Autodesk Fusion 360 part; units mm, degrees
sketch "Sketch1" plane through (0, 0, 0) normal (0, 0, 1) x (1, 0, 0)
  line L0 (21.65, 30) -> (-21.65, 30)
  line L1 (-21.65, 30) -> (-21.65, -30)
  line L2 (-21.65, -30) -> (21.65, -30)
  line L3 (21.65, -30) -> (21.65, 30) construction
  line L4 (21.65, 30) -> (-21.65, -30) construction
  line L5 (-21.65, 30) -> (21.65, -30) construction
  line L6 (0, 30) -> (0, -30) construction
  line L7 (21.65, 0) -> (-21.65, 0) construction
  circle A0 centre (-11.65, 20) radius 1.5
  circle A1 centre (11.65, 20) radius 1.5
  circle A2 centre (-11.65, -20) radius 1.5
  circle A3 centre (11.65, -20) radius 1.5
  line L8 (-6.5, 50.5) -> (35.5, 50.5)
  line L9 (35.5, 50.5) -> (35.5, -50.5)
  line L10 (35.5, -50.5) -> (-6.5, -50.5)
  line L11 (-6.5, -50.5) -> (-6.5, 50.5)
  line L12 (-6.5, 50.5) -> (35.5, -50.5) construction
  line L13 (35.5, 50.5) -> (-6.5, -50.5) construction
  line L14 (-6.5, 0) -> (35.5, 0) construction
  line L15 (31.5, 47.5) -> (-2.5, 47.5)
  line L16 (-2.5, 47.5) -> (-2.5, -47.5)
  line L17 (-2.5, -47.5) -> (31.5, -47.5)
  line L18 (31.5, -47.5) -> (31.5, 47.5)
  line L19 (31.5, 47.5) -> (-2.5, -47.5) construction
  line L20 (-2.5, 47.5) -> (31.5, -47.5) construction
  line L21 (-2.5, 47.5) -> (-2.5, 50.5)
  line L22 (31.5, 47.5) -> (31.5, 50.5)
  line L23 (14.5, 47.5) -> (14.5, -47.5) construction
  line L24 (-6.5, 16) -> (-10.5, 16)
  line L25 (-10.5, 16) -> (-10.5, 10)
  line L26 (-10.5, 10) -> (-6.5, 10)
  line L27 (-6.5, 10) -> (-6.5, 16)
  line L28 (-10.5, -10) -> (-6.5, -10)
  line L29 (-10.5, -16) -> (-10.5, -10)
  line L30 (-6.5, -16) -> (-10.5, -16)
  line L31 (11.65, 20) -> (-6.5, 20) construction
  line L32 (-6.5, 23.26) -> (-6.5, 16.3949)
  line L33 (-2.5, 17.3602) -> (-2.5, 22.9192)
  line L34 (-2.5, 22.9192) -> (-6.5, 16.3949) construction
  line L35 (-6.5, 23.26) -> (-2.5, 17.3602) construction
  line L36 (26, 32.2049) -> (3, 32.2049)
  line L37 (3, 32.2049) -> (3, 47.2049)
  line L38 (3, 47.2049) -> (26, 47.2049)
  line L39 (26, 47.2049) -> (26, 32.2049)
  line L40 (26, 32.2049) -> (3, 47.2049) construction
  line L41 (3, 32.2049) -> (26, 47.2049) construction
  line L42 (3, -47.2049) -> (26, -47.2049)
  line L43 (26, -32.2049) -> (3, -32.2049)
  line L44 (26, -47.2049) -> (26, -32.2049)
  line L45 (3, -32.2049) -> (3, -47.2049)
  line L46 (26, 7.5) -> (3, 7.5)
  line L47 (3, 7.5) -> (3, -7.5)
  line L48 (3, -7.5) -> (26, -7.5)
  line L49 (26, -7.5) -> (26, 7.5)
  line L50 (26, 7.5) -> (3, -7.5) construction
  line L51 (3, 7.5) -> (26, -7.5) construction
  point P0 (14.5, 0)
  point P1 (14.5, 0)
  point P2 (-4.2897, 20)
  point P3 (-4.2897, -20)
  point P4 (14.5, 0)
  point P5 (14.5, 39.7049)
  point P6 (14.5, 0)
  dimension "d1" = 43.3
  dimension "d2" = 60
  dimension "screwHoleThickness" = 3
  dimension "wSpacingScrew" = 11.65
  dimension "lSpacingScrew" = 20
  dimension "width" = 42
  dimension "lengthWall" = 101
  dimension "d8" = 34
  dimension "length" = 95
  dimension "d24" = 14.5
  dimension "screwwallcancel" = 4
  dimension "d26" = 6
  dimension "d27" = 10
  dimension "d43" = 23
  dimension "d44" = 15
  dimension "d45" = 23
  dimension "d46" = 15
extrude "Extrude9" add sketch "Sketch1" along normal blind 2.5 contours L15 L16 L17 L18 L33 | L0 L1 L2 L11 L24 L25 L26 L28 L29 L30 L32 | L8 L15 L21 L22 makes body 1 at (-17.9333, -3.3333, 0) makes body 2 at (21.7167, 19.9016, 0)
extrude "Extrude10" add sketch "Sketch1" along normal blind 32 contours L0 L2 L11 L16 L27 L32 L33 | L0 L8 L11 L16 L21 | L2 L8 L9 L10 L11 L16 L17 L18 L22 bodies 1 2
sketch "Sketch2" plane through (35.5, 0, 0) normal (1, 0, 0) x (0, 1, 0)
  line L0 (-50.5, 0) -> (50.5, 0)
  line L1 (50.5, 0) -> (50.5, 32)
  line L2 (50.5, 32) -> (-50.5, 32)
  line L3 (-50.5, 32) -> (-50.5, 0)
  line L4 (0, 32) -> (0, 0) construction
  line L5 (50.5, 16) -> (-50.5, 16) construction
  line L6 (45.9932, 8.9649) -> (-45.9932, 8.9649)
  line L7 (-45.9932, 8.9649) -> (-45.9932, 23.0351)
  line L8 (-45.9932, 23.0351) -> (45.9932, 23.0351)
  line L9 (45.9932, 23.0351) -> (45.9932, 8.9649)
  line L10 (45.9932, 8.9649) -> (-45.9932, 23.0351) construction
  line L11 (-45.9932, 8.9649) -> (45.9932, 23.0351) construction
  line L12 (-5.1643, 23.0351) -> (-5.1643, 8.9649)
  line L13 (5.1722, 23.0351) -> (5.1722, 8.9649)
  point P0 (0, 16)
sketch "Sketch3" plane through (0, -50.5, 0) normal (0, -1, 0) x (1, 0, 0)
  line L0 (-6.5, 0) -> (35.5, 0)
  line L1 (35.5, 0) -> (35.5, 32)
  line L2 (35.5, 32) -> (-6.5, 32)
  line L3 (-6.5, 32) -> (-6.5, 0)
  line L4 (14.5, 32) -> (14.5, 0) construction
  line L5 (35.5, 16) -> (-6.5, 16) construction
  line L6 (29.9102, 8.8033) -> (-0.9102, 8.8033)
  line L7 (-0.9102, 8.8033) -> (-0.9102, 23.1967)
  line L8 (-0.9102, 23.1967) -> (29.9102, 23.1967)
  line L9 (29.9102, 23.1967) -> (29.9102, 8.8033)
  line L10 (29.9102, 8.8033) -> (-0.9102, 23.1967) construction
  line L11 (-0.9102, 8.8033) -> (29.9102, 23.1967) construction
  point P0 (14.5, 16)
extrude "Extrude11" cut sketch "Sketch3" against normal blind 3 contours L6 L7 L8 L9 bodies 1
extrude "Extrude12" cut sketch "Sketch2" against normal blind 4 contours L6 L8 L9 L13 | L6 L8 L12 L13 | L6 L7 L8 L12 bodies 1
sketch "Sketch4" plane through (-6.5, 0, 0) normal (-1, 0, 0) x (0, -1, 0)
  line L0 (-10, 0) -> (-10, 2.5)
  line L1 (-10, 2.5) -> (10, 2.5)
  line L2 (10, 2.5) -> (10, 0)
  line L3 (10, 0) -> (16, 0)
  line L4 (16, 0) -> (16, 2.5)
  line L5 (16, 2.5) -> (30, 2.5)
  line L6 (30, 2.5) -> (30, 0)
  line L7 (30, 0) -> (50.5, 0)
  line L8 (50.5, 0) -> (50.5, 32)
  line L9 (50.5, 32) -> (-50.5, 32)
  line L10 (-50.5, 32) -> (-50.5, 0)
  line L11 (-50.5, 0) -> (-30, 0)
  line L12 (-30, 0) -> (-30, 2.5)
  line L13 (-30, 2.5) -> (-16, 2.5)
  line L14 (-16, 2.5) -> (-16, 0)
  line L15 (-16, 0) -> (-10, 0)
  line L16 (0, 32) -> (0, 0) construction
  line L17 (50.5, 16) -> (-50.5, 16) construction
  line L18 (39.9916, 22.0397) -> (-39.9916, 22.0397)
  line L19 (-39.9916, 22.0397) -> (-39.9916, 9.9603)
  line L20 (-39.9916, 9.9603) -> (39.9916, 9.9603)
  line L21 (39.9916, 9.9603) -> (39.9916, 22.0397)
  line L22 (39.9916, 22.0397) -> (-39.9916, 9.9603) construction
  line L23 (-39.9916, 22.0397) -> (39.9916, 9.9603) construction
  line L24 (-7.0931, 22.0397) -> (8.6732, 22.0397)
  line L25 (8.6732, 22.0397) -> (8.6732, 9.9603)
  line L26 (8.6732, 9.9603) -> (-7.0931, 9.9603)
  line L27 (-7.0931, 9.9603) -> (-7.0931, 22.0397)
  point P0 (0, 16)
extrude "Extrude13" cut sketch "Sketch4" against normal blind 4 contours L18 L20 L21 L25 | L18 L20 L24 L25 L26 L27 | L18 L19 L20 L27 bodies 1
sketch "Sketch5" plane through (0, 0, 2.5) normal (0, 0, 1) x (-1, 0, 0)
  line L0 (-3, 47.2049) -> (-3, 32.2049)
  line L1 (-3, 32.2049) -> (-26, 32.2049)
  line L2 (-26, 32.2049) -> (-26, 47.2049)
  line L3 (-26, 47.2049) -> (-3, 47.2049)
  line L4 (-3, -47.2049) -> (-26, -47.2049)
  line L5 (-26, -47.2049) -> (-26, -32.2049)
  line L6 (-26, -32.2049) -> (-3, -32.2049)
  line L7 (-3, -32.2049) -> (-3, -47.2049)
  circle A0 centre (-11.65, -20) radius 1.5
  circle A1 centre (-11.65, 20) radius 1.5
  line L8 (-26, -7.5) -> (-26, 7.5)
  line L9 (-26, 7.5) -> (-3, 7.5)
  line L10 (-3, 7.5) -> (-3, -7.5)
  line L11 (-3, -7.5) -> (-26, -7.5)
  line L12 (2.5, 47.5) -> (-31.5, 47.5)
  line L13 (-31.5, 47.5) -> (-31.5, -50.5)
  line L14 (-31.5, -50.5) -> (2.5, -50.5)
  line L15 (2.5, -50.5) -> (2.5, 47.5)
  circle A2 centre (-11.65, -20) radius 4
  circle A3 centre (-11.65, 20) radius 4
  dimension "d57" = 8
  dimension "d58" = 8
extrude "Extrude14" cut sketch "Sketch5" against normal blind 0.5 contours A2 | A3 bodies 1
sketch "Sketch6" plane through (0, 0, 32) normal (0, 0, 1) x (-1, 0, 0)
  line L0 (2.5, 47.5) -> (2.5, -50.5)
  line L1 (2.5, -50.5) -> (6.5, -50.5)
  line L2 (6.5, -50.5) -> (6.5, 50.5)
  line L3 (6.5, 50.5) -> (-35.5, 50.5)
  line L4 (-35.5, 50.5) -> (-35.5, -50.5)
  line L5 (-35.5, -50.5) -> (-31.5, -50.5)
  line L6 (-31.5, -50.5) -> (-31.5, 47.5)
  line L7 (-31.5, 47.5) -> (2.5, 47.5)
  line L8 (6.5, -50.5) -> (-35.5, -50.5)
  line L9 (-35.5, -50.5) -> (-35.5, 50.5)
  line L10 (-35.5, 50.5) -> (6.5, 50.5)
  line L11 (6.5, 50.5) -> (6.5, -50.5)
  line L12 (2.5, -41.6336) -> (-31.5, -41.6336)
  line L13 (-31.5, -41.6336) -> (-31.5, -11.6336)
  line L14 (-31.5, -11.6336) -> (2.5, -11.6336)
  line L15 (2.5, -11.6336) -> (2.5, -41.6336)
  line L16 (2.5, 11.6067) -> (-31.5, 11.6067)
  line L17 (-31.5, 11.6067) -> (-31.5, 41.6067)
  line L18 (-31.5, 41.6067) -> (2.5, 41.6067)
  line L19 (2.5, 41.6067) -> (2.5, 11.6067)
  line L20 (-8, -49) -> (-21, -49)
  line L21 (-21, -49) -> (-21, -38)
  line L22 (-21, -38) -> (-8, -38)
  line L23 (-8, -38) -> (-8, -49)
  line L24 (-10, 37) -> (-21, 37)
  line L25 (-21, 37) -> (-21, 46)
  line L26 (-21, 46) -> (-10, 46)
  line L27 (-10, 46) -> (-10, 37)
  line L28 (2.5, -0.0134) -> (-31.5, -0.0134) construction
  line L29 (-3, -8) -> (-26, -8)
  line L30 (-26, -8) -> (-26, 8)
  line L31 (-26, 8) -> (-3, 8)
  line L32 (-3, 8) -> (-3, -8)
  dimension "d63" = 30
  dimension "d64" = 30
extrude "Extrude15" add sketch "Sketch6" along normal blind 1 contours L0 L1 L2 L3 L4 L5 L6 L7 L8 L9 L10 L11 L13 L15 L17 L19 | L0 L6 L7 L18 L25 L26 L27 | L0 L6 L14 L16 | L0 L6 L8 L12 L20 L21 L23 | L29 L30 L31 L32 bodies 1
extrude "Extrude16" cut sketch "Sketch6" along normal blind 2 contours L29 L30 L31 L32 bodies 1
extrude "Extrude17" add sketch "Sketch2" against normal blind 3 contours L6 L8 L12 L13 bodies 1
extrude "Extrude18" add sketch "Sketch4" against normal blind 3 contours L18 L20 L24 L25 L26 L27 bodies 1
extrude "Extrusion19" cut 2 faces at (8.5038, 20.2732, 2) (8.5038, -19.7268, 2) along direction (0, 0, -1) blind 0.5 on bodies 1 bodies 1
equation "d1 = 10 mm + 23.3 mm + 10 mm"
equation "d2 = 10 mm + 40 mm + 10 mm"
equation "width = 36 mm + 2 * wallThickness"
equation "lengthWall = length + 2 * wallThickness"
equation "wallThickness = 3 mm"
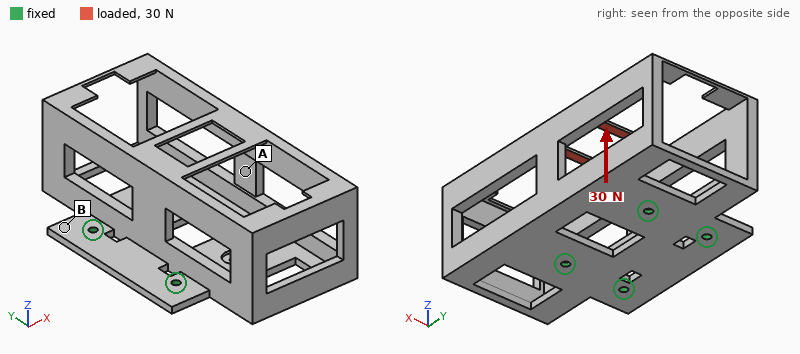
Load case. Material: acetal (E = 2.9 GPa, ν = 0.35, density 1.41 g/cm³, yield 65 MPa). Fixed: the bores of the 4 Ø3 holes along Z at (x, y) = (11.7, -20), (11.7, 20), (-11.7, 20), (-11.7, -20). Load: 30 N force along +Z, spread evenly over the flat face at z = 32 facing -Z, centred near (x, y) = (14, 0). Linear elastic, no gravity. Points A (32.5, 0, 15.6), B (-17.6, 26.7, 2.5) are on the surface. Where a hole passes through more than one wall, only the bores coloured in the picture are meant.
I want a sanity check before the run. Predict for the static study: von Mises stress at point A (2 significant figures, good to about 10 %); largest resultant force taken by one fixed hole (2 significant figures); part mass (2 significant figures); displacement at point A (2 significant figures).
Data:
3.3 MPa
16 N
41 g
0.26 mm
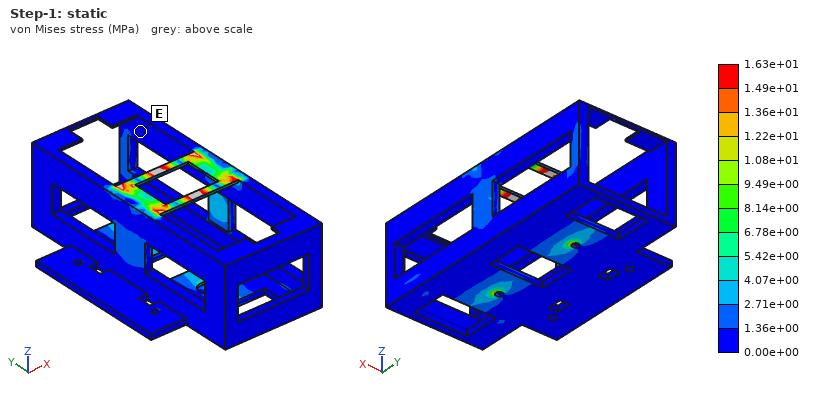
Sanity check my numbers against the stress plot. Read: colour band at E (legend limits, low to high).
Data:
0.00e+00 to 1.36e+00 MPa
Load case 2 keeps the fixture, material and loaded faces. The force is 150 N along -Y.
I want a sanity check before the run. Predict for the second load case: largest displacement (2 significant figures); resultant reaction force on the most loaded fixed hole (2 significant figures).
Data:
1.2 mm
73 N
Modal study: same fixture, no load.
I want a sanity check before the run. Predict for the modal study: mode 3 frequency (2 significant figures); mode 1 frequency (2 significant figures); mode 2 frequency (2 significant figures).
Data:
540 Hz
280 Hz
390 Hz
